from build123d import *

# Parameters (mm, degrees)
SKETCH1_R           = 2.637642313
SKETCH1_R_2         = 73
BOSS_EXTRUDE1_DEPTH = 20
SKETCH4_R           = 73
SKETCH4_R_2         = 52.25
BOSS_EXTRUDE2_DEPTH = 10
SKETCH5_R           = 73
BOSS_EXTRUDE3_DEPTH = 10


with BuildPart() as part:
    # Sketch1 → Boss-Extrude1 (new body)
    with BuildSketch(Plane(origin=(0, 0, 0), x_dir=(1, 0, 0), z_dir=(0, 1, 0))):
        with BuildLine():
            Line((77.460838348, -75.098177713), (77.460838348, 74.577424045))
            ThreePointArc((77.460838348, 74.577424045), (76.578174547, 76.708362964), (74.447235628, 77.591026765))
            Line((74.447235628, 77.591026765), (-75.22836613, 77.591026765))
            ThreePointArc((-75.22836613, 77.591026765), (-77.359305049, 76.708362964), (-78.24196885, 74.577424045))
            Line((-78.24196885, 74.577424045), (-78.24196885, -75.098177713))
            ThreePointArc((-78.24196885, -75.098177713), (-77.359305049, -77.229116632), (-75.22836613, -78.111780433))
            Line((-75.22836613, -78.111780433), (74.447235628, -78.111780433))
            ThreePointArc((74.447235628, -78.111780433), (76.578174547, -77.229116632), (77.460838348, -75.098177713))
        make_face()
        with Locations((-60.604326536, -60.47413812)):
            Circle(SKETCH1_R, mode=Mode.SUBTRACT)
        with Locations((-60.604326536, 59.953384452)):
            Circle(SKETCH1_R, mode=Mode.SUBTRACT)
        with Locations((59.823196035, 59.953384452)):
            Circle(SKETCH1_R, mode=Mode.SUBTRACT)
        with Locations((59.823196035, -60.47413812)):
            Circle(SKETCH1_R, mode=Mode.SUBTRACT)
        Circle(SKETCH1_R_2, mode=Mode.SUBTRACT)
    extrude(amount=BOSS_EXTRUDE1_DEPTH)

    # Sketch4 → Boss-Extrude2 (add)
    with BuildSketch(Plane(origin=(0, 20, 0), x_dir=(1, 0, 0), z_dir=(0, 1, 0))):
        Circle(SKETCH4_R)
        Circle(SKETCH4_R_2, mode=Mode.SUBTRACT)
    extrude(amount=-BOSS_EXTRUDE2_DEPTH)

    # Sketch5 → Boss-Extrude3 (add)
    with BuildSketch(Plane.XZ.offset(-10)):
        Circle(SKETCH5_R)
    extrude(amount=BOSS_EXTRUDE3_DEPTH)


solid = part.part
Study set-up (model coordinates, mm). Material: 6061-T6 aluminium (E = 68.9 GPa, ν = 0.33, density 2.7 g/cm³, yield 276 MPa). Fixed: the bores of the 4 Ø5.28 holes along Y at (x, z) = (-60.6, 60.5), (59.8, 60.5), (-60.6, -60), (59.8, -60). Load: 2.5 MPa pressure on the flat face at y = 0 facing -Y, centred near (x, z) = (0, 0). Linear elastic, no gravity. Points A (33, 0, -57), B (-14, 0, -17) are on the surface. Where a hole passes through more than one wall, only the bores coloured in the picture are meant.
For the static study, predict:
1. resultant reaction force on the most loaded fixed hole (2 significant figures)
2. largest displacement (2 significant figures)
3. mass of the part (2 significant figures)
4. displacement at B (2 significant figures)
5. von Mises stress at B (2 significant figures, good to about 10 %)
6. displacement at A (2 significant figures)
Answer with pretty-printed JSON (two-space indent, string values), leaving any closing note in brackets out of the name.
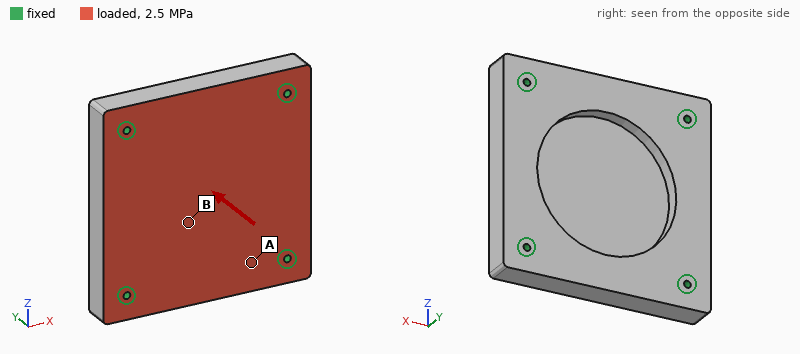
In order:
{
  "resultant reaction force on the most loaded fixed hole": "16 kN",
  "largest displacement": "0.22 mm",
  "mass of the part": "1.1 kg",
  "displacement at B": "0.19 mm",
  "von Mises stress at B": "56 MPa",
  "displacement at A": "0.061 mm"
}
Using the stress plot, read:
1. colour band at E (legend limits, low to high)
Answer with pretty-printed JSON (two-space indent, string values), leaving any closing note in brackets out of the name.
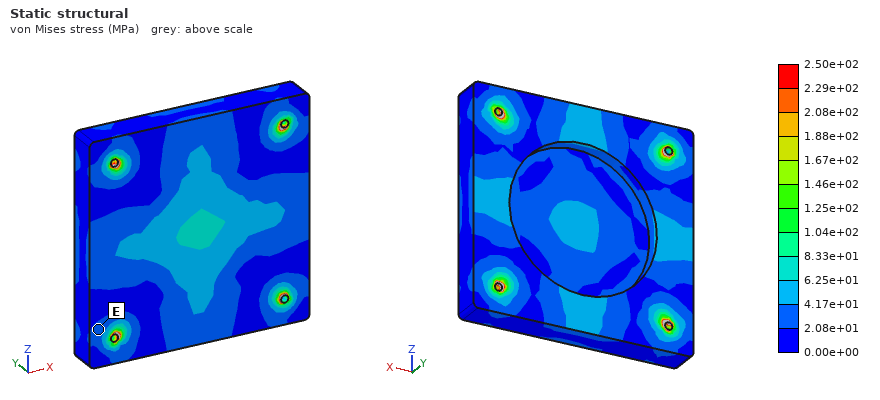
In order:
{
  "colour band at E": "2.08e+01 to 4.17e+01 MPa"
}
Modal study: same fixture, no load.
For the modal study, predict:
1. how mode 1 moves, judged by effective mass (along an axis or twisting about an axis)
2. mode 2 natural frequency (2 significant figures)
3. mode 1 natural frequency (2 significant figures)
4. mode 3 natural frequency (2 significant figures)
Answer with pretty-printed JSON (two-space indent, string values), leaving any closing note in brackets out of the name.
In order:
{
  "how mode 1 moves, judged by effective mass": "along Y",
  "mode 2 natural frequency": "5500 Hz",
  "mode 1 natural frequency": "3900 Hz",
  "mode 3 natural frequency": "5500 Hz"
}
